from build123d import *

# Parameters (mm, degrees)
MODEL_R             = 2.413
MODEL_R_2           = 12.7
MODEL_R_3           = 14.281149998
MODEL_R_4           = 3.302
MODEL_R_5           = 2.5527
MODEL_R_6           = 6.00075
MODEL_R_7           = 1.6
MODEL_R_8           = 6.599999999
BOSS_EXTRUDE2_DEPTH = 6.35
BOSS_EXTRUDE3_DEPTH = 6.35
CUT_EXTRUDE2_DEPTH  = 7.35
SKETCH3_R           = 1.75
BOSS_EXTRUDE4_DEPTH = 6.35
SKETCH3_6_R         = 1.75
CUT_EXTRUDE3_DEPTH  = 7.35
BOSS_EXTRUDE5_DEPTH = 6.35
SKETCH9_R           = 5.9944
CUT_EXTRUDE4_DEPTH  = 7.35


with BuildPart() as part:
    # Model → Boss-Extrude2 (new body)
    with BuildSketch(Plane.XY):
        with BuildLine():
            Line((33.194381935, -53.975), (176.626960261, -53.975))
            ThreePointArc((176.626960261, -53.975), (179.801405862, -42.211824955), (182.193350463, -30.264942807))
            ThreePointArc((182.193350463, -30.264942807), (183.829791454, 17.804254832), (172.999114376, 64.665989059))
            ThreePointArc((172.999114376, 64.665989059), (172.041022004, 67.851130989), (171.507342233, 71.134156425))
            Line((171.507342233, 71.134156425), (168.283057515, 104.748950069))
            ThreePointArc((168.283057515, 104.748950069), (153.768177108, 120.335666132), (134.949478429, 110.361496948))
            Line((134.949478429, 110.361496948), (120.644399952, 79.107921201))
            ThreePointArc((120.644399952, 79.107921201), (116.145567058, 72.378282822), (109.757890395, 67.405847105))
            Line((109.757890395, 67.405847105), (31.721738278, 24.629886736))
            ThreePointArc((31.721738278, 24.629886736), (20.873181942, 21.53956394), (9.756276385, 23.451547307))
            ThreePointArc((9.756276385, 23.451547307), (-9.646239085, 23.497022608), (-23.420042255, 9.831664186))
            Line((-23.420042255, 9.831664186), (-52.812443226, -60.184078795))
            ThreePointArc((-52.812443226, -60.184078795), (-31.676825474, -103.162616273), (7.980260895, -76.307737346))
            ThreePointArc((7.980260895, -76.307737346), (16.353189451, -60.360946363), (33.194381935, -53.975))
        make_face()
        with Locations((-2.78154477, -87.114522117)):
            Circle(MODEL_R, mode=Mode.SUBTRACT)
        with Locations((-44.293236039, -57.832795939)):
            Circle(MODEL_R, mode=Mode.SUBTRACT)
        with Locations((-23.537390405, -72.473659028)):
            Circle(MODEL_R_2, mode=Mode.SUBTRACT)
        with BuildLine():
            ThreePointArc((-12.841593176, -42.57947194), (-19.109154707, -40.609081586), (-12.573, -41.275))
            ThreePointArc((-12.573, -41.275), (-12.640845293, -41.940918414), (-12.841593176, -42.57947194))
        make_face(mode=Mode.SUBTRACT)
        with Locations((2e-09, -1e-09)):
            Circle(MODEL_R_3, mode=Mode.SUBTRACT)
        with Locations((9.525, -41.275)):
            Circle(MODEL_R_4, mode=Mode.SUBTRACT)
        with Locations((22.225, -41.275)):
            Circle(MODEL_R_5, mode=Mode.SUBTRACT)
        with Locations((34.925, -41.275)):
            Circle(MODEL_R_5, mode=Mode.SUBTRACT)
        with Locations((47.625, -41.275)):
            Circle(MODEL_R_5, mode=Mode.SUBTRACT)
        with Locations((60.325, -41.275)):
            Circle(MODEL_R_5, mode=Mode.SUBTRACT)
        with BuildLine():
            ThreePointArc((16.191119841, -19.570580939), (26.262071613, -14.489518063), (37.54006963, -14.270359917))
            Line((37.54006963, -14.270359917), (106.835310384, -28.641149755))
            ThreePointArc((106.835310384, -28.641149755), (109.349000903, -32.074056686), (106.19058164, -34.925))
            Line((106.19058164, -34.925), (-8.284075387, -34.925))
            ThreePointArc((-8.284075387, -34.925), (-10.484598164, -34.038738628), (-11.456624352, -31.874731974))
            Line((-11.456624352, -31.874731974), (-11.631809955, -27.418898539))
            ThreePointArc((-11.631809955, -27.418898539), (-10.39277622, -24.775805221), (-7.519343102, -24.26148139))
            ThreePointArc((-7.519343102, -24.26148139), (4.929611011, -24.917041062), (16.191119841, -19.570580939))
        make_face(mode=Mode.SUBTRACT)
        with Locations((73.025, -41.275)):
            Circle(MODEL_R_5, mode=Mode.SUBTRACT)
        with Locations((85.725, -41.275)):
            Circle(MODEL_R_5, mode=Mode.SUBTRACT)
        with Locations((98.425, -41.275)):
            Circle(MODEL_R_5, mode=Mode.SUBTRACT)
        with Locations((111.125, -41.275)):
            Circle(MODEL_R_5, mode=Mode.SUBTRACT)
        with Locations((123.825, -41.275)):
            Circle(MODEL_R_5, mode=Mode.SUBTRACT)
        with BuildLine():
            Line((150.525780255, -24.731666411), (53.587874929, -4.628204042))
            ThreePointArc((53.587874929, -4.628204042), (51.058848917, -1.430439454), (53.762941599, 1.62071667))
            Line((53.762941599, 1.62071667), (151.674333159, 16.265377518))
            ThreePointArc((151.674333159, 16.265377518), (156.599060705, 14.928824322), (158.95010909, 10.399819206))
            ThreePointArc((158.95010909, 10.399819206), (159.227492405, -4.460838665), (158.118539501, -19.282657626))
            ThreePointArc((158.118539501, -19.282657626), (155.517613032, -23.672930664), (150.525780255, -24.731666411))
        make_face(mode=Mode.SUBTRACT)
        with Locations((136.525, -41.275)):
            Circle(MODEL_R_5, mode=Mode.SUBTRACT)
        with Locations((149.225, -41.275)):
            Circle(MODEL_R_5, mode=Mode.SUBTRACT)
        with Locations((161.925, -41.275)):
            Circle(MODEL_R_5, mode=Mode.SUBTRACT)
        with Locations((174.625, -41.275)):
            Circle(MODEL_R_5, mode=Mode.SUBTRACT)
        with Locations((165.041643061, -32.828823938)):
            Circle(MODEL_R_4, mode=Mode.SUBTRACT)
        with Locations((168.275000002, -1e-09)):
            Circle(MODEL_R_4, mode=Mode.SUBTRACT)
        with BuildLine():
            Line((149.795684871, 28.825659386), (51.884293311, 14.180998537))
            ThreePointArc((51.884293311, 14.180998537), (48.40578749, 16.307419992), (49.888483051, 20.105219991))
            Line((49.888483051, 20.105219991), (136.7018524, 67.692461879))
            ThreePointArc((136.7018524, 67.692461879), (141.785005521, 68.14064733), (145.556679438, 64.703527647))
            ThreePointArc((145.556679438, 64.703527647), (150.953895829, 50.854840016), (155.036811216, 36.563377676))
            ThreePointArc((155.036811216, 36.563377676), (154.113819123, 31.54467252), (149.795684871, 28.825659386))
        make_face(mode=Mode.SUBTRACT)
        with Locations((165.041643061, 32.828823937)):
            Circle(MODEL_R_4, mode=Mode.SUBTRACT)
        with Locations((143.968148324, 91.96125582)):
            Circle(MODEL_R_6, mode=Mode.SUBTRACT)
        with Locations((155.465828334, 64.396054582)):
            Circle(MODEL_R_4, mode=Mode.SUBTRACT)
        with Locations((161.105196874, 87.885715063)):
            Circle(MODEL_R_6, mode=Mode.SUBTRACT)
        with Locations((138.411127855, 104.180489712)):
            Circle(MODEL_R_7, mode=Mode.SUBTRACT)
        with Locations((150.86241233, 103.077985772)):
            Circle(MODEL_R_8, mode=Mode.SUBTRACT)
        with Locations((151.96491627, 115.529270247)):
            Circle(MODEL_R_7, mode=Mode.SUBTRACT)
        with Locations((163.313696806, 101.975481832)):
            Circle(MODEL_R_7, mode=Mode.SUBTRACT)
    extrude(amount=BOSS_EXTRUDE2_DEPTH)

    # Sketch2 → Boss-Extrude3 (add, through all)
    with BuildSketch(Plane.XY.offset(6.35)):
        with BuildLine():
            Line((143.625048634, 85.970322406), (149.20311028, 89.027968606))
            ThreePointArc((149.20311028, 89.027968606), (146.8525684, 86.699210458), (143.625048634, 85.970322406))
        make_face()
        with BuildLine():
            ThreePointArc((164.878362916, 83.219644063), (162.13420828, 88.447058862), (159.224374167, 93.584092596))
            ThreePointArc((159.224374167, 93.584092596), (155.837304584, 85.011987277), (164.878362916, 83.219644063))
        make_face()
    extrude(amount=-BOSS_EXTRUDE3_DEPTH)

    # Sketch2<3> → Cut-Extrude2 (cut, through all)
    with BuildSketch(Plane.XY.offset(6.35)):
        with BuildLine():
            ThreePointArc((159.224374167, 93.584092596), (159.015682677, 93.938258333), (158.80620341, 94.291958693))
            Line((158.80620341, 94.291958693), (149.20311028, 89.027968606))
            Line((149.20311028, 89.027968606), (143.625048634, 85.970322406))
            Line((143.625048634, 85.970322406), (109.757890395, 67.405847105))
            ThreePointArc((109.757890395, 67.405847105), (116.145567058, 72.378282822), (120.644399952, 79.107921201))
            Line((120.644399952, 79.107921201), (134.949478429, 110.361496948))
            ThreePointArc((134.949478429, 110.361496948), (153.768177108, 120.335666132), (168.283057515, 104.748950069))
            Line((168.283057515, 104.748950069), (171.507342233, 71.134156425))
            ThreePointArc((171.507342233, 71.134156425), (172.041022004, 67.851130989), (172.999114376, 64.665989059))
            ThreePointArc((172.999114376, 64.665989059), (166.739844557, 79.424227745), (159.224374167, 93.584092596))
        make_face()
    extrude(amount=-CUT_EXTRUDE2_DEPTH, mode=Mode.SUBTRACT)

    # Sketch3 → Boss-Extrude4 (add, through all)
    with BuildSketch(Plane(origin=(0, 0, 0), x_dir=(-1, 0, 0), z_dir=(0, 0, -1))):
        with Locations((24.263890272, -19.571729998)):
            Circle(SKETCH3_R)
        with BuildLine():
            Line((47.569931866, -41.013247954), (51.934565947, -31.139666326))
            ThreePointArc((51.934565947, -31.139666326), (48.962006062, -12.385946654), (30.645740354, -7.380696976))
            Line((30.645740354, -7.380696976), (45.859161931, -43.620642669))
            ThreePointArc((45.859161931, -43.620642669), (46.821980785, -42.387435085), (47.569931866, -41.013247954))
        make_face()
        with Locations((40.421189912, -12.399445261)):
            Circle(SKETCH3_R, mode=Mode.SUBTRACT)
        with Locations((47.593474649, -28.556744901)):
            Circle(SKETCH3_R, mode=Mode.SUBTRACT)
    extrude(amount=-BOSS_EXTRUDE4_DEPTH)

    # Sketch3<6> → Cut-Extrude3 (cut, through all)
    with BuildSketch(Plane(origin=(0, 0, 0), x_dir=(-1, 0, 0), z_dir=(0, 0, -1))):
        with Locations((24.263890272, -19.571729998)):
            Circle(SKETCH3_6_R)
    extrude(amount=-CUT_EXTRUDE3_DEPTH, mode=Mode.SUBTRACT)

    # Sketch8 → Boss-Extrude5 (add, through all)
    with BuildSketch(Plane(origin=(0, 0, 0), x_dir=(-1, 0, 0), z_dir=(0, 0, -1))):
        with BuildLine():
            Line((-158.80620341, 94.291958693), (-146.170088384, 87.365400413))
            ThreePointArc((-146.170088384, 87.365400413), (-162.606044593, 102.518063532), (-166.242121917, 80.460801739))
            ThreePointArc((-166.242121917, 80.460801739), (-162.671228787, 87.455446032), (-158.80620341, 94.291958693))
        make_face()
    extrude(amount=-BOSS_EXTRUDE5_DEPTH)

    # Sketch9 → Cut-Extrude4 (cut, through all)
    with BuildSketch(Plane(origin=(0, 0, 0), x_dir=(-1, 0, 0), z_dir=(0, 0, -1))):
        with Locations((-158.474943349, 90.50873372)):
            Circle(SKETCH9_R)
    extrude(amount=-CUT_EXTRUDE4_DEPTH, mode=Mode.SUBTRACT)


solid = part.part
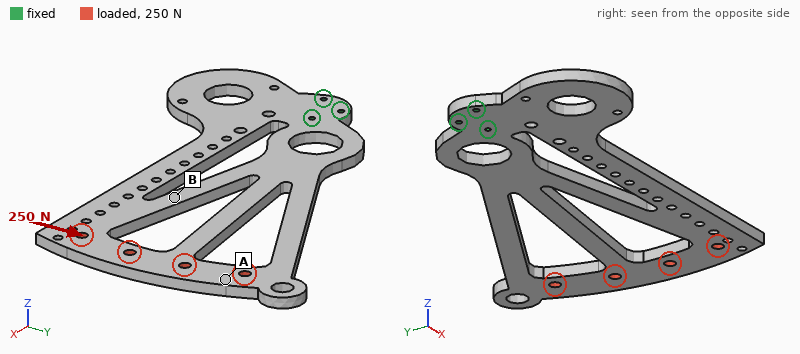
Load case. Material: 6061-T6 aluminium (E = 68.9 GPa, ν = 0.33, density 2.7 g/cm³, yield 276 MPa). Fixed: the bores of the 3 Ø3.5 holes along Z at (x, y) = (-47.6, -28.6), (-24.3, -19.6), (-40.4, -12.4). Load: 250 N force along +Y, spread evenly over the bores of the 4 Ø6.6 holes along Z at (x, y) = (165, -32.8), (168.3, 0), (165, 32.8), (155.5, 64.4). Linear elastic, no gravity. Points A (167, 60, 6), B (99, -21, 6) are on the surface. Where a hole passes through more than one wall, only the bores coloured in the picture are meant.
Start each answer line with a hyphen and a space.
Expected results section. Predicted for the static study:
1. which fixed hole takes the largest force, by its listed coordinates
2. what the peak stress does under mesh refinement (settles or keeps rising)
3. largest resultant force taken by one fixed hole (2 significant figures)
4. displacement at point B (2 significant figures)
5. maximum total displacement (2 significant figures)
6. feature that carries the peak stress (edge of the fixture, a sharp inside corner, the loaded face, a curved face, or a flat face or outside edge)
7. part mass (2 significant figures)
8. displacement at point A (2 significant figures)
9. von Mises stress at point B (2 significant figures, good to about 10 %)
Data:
- (-24.3, -19.6)
- keeps rising
- 1.7 kN
- 0.14 mm
- 0.27 mm
- edge of the fixture
- 300 g
- 0.25 mm
- 6.2 MPa
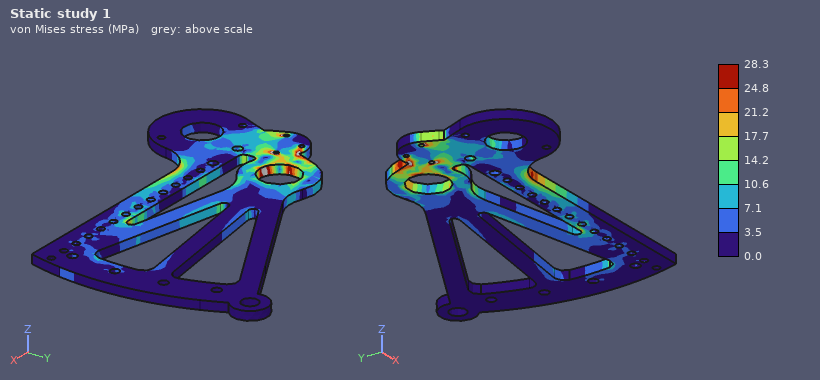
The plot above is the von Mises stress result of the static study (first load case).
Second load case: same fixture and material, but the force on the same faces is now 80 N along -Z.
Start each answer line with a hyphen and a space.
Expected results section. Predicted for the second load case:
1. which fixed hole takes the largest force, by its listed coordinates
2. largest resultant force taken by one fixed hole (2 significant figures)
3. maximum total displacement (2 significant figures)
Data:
- (-24.3, -19.6)
- 610 N
- 3.5 mm
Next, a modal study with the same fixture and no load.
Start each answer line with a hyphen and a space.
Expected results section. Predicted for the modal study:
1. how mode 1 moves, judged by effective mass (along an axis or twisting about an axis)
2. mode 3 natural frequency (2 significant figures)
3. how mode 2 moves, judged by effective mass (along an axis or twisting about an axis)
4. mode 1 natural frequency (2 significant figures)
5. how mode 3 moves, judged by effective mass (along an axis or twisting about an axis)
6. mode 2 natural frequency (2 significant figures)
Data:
- along Z
- 470 Hz
- twisting about X
- 82 Hz
- along Y
- 240 Hz
